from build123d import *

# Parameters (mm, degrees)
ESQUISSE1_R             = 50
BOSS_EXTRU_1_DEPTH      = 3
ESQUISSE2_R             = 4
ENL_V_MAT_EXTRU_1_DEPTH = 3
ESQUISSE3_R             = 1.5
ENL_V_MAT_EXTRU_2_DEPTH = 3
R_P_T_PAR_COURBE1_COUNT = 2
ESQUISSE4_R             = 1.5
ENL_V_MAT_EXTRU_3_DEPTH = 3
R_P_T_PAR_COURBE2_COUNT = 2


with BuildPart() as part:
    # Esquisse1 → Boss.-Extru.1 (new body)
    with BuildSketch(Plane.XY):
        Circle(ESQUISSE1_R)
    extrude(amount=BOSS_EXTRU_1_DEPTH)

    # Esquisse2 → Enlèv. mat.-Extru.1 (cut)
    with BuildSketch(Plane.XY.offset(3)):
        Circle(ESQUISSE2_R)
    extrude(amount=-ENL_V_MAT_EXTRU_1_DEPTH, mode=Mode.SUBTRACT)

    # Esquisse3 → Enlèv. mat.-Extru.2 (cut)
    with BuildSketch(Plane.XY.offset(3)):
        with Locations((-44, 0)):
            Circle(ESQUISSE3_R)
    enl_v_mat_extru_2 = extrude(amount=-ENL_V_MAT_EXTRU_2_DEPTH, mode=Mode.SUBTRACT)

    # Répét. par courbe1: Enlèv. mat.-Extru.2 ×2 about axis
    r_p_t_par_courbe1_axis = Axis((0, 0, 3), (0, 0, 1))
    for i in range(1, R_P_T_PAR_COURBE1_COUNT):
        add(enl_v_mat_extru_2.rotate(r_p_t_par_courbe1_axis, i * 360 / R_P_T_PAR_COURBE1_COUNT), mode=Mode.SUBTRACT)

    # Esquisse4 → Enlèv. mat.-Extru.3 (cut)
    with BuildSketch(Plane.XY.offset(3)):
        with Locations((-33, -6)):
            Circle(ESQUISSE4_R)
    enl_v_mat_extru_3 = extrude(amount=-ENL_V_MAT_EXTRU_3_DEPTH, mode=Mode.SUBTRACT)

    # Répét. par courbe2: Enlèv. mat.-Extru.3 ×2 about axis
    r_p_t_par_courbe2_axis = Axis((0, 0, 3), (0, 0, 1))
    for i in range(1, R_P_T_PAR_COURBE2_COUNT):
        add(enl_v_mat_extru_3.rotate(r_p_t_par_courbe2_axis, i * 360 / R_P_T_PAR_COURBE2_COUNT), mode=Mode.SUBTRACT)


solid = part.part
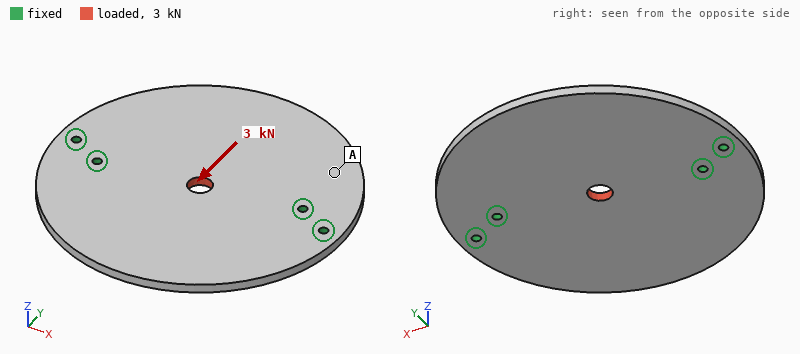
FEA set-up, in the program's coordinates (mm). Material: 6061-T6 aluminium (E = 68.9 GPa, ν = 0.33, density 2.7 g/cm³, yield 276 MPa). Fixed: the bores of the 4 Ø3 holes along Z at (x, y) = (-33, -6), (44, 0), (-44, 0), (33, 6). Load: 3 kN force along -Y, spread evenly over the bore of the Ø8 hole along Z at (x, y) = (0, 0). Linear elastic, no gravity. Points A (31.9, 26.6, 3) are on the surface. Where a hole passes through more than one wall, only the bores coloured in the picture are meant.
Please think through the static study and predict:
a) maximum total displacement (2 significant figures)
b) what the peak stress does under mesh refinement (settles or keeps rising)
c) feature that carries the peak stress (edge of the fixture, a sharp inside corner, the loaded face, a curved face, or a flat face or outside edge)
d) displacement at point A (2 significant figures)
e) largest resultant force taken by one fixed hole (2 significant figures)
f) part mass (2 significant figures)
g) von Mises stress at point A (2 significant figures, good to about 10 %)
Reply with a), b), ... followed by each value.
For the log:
a) 16 µm
b) keeps rising
c) edge of the fixture
d) 4.1 µm
e) 1.1 kN
f) 63 g
g) 8.2 MPa
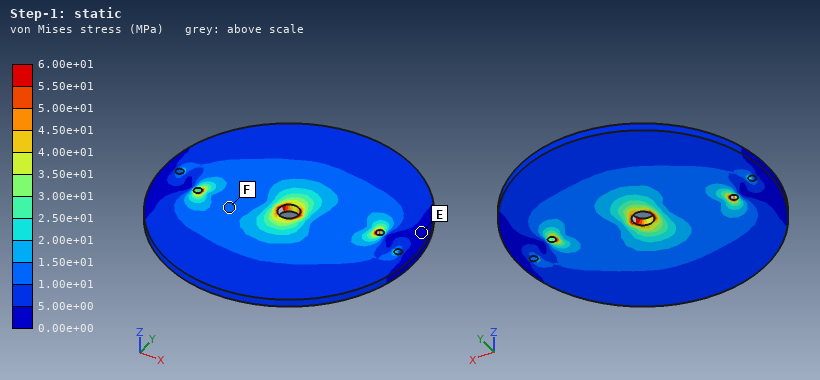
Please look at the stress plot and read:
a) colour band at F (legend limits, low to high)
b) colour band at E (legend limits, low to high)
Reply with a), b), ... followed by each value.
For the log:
a) 1.00e+01 to 1.50e+01 MPa
b) 0.00e+00 to 5.00e+00 MPa
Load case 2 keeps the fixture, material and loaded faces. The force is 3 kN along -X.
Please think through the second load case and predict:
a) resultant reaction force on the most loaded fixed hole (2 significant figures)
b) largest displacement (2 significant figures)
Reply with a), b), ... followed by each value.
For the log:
a) 1.0 kN
b) 12 µm
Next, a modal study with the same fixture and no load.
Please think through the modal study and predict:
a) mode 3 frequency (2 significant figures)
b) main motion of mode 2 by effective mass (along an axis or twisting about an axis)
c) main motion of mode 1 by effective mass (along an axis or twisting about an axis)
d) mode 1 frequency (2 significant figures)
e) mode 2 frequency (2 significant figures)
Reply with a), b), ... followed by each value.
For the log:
a) 2700 Hz
b) along Z
c) twisting about X
d) 980 Hz
e) 1200 Hz
